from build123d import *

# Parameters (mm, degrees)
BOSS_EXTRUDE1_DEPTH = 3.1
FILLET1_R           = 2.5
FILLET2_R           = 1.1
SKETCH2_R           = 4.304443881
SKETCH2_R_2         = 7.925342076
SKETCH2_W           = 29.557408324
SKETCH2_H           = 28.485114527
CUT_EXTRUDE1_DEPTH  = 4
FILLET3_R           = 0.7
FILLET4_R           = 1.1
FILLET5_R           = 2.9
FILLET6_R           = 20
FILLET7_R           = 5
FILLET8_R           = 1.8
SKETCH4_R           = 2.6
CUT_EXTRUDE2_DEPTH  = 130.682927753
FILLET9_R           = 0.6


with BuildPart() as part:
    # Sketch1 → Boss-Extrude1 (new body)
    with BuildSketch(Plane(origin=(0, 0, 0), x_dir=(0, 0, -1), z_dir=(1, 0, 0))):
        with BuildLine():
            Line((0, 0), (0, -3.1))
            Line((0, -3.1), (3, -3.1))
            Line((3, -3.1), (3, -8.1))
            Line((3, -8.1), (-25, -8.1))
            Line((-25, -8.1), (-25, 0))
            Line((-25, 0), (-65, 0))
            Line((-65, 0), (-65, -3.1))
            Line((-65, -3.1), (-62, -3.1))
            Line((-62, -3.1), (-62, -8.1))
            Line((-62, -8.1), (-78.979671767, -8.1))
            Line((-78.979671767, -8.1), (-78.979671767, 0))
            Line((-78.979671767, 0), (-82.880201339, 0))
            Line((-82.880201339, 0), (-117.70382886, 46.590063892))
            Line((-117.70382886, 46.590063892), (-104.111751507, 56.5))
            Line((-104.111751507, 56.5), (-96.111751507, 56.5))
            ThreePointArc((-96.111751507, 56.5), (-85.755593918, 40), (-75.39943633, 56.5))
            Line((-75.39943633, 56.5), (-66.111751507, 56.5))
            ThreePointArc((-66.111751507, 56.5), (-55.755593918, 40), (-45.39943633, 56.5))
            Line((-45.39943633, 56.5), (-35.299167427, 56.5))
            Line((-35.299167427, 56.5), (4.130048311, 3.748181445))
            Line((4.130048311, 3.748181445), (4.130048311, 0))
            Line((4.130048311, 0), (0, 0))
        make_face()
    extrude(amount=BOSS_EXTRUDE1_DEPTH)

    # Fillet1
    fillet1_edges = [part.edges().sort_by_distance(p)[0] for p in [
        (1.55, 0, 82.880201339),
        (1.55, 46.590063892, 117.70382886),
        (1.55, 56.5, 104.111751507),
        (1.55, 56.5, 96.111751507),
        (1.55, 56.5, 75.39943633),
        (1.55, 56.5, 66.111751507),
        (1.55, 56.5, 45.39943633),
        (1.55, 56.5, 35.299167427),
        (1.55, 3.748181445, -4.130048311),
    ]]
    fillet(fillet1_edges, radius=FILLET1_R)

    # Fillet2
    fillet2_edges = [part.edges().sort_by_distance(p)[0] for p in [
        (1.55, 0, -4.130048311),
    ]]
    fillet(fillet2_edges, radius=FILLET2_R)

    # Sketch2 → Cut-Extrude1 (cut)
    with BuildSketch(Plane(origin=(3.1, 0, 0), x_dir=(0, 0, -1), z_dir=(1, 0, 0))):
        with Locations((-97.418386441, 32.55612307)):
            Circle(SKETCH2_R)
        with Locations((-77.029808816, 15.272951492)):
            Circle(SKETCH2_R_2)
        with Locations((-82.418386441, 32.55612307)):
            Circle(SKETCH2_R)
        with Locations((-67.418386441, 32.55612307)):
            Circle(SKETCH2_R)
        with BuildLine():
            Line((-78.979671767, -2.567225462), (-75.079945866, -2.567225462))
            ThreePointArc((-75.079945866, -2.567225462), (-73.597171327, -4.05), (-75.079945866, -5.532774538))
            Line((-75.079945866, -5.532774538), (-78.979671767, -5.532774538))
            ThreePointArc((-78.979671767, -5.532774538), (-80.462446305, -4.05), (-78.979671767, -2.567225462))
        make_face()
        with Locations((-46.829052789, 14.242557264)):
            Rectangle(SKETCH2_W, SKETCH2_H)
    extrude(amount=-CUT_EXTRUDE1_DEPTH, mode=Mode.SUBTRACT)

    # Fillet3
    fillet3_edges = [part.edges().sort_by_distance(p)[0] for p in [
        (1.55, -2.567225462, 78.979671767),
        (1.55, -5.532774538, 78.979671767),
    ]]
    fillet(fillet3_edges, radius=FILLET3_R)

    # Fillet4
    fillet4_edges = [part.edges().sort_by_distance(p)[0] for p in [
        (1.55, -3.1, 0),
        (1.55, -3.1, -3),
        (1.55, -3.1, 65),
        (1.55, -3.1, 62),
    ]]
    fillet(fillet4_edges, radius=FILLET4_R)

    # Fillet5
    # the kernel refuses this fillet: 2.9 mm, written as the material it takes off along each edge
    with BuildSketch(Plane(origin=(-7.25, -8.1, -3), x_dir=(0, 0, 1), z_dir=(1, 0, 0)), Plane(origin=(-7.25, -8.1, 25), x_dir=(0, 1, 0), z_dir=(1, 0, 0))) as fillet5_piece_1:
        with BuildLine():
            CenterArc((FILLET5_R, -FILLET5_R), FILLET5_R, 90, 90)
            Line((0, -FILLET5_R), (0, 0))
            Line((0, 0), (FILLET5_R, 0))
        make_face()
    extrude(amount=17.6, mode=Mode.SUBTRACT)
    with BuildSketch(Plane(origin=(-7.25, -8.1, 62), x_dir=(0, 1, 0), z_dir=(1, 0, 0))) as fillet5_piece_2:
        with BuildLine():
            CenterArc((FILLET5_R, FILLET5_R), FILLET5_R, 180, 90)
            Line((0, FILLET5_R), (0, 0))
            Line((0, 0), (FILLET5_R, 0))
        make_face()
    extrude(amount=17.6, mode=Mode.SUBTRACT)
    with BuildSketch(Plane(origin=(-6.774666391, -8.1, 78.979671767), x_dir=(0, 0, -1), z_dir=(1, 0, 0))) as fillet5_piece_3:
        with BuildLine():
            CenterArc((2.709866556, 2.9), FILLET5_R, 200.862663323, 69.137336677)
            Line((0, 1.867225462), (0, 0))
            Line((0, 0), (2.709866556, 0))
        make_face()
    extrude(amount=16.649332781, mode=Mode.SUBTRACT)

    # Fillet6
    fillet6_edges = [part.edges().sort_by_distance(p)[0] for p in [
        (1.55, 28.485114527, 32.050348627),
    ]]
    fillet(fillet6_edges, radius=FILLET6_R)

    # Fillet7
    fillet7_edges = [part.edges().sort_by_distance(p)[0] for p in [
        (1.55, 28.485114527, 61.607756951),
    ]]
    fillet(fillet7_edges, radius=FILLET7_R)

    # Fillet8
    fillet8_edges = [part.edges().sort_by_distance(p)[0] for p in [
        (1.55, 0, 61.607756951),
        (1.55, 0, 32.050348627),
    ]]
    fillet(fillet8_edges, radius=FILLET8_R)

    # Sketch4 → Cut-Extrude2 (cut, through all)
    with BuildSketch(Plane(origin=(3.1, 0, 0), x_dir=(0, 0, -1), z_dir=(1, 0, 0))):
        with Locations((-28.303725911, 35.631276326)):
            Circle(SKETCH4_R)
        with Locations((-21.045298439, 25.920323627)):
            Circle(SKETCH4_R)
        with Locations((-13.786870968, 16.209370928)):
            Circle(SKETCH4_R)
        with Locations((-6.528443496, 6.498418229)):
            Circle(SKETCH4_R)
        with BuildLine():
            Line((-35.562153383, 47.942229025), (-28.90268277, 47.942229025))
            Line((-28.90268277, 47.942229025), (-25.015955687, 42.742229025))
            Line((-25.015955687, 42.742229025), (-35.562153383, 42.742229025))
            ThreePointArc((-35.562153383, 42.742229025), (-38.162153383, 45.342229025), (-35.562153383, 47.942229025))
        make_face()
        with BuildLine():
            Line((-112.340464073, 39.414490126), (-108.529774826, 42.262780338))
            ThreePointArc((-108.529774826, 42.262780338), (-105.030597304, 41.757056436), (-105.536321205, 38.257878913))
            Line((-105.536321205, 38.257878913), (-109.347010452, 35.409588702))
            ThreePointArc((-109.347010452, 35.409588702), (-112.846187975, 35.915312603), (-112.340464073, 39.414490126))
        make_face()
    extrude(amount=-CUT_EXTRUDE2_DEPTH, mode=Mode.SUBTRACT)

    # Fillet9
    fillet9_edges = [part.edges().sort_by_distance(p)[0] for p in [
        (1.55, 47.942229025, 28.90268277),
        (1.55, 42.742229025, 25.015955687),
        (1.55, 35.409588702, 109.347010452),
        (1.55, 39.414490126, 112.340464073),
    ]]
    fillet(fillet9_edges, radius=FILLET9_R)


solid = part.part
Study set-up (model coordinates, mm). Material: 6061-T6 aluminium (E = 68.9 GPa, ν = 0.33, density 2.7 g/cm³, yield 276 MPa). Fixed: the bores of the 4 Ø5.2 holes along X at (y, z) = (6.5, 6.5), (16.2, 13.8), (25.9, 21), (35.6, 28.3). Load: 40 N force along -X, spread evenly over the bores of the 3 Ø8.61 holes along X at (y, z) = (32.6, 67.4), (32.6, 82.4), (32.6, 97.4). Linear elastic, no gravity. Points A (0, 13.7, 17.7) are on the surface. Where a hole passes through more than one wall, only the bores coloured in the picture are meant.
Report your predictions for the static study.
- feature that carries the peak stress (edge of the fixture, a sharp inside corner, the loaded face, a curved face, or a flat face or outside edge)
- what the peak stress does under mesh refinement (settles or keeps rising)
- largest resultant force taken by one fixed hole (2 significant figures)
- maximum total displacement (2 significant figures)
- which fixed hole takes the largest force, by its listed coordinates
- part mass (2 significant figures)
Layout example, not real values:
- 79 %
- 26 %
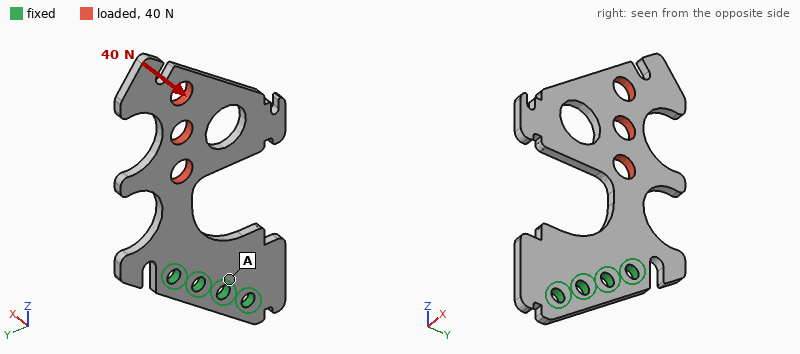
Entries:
- edge of the fixture
- keeps rising
- 85 N
- 1.4 mm
- (35.6, 28.3)
- 28 g
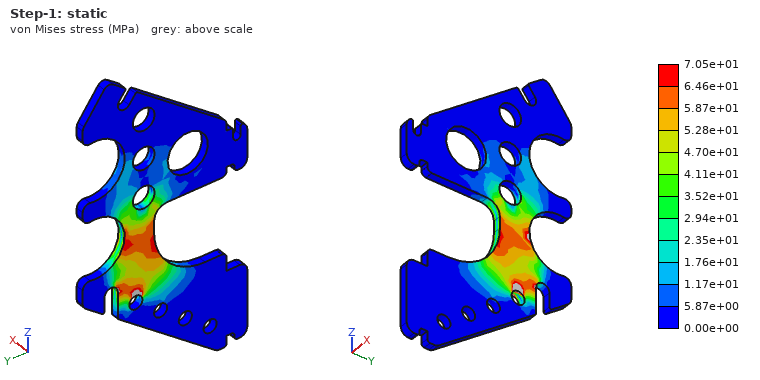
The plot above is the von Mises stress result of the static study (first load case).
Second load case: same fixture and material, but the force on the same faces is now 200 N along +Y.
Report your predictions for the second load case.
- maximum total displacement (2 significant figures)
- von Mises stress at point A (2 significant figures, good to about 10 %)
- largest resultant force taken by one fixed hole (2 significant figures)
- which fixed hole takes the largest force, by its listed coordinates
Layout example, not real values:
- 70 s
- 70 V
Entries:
- 0.34 mm
- 6.4 MPa
- 610 N
- (35.6, 28.3)
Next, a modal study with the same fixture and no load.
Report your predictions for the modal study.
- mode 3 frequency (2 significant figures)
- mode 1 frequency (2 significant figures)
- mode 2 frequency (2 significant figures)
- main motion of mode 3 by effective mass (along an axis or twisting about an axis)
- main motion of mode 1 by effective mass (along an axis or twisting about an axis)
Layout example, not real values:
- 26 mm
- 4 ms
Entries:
- 1200 Hz
- 300 Hz
- 650 Hz
- along Y
- along X
